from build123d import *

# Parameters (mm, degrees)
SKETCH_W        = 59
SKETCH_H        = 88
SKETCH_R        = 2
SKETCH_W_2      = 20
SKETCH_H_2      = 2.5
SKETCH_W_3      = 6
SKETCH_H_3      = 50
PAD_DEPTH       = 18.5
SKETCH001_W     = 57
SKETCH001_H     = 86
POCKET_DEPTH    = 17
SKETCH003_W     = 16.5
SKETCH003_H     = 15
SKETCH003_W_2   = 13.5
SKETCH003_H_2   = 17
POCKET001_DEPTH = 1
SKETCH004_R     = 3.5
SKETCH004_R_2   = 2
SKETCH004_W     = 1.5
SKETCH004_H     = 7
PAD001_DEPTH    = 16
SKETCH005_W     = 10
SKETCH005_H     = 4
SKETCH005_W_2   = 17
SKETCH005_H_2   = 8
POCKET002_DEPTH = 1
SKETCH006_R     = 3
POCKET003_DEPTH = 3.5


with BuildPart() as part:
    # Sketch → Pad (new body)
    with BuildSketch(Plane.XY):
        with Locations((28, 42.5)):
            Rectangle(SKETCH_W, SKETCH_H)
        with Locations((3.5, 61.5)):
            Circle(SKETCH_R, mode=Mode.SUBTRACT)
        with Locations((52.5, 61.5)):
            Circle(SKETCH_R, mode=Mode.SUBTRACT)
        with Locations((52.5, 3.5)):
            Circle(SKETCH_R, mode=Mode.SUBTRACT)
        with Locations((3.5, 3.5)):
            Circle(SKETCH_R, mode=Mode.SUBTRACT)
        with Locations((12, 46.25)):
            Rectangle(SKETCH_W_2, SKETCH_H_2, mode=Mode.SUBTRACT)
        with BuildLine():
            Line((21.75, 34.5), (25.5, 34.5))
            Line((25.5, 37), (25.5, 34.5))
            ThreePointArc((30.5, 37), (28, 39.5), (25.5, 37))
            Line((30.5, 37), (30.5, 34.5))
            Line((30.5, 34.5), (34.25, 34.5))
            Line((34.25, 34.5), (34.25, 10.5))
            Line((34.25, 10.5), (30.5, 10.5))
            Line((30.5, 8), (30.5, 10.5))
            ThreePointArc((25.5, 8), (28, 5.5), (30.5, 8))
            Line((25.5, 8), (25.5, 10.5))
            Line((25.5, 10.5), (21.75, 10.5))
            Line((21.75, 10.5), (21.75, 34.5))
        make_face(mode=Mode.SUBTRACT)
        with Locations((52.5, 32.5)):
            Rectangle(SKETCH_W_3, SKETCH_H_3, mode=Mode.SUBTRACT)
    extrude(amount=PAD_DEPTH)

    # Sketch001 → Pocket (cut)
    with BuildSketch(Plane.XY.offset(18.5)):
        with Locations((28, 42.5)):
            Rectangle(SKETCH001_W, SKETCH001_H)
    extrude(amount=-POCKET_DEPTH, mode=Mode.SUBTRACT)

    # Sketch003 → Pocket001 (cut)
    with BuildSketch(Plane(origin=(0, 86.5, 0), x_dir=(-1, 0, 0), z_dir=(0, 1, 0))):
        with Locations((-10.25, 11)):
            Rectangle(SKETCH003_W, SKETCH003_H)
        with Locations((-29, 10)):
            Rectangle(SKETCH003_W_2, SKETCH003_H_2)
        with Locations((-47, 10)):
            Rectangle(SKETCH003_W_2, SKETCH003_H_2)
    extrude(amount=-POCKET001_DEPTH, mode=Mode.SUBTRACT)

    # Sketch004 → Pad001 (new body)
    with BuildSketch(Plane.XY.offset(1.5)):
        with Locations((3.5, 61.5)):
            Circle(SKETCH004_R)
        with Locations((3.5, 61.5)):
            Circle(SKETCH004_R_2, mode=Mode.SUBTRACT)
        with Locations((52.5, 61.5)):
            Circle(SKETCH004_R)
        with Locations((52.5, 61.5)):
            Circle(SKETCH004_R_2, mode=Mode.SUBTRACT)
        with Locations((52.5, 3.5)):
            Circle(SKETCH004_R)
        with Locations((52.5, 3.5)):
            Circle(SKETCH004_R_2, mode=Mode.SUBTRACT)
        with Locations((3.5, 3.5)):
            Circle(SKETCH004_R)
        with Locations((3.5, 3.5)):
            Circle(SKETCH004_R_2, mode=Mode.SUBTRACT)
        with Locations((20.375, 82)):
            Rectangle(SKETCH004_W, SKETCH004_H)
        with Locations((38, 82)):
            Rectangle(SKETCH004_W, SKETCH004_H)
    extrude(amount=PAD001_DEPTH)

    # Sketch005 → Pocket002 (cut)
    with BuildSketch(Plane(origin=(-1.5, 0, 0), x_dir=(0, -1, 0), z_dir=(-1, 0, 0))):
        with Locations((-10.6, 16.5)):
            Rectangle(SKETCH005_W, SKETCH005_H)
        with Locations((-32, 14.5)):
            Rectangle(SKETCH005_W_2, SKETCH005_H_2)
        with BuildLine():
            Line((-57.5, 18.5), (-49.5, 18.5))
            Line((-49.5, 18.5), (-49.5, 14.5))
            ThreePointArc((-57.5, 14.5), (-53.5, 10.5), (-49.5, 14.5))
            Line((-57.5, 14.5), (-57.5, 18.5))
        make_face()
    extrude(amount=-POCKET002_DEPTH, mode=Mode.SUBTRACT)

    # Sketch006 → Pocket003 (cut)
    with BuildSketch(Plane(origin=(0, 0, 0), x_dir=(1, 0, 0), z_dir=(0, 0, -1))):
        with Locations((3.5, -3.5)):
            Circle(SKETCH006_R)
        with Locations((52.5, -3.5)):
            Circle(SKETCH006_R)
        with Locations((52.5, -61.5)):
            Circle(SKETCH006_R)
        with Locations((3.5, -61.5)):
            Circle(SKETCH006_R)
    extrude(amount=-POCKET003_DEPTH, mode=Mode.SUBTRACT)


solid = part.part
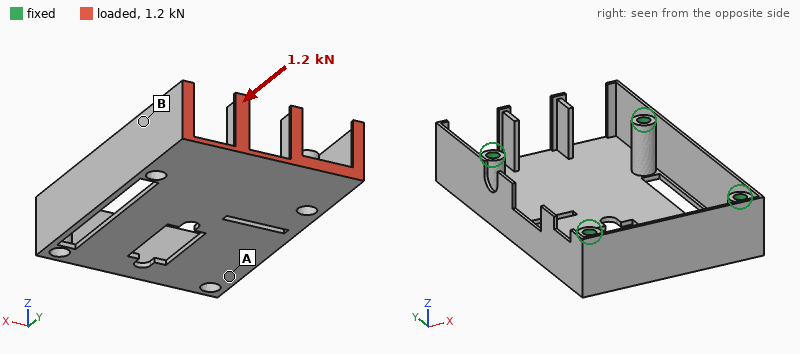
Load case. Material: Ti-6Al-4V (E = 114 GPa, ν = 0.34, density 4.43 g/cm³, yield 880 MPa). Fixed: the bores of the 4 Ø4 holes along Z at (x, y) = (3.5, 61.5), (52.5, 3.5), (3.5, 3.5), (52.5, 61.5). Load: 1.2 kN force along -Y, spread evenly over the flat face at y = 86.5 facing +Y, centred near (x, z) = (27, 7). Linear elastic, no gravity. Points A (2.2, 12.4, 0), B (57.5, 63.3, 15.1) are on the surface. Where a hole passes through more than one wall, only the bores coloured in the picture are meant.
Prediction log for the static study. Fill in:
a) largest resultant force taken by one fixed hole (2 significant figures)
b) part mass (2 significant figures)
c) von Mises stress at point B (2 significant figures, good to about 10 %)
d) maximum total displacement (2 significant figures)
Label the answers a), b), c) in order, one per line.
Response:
a) 370 N
b) 55 g
c) 57 MPa
d) 0.75 mm
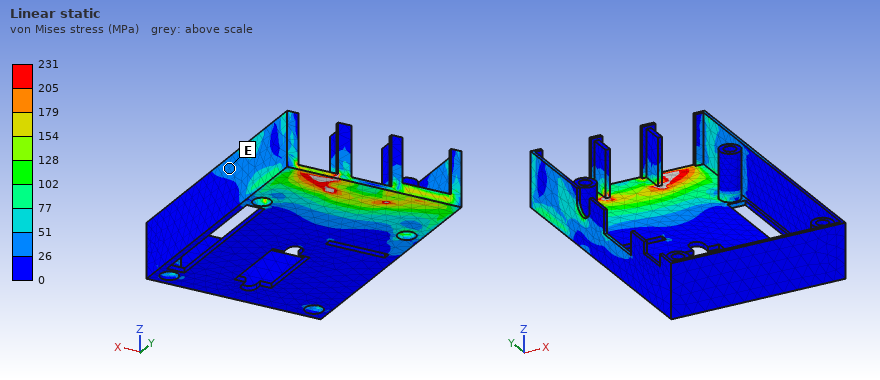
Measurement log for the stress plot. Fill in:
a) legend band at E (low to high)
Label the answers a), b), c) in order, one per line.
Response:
a) 26 to 51 MPa
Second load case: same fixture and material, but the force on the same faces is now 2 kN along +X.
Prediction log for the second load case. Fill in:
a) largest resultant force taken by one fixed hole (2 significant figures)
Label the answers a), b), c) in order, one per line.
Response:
a) 1.4 kN
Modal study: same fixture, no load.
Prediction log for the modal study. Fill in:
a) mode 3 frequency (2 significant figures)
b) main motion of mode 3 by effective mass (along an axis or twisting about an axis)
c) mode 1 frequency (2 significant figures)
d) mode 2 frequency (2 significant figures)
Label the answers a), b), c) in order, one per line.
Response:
a) 1900 Hz
b) along Z
c) 1500 Hz
d) 1500 Hz
